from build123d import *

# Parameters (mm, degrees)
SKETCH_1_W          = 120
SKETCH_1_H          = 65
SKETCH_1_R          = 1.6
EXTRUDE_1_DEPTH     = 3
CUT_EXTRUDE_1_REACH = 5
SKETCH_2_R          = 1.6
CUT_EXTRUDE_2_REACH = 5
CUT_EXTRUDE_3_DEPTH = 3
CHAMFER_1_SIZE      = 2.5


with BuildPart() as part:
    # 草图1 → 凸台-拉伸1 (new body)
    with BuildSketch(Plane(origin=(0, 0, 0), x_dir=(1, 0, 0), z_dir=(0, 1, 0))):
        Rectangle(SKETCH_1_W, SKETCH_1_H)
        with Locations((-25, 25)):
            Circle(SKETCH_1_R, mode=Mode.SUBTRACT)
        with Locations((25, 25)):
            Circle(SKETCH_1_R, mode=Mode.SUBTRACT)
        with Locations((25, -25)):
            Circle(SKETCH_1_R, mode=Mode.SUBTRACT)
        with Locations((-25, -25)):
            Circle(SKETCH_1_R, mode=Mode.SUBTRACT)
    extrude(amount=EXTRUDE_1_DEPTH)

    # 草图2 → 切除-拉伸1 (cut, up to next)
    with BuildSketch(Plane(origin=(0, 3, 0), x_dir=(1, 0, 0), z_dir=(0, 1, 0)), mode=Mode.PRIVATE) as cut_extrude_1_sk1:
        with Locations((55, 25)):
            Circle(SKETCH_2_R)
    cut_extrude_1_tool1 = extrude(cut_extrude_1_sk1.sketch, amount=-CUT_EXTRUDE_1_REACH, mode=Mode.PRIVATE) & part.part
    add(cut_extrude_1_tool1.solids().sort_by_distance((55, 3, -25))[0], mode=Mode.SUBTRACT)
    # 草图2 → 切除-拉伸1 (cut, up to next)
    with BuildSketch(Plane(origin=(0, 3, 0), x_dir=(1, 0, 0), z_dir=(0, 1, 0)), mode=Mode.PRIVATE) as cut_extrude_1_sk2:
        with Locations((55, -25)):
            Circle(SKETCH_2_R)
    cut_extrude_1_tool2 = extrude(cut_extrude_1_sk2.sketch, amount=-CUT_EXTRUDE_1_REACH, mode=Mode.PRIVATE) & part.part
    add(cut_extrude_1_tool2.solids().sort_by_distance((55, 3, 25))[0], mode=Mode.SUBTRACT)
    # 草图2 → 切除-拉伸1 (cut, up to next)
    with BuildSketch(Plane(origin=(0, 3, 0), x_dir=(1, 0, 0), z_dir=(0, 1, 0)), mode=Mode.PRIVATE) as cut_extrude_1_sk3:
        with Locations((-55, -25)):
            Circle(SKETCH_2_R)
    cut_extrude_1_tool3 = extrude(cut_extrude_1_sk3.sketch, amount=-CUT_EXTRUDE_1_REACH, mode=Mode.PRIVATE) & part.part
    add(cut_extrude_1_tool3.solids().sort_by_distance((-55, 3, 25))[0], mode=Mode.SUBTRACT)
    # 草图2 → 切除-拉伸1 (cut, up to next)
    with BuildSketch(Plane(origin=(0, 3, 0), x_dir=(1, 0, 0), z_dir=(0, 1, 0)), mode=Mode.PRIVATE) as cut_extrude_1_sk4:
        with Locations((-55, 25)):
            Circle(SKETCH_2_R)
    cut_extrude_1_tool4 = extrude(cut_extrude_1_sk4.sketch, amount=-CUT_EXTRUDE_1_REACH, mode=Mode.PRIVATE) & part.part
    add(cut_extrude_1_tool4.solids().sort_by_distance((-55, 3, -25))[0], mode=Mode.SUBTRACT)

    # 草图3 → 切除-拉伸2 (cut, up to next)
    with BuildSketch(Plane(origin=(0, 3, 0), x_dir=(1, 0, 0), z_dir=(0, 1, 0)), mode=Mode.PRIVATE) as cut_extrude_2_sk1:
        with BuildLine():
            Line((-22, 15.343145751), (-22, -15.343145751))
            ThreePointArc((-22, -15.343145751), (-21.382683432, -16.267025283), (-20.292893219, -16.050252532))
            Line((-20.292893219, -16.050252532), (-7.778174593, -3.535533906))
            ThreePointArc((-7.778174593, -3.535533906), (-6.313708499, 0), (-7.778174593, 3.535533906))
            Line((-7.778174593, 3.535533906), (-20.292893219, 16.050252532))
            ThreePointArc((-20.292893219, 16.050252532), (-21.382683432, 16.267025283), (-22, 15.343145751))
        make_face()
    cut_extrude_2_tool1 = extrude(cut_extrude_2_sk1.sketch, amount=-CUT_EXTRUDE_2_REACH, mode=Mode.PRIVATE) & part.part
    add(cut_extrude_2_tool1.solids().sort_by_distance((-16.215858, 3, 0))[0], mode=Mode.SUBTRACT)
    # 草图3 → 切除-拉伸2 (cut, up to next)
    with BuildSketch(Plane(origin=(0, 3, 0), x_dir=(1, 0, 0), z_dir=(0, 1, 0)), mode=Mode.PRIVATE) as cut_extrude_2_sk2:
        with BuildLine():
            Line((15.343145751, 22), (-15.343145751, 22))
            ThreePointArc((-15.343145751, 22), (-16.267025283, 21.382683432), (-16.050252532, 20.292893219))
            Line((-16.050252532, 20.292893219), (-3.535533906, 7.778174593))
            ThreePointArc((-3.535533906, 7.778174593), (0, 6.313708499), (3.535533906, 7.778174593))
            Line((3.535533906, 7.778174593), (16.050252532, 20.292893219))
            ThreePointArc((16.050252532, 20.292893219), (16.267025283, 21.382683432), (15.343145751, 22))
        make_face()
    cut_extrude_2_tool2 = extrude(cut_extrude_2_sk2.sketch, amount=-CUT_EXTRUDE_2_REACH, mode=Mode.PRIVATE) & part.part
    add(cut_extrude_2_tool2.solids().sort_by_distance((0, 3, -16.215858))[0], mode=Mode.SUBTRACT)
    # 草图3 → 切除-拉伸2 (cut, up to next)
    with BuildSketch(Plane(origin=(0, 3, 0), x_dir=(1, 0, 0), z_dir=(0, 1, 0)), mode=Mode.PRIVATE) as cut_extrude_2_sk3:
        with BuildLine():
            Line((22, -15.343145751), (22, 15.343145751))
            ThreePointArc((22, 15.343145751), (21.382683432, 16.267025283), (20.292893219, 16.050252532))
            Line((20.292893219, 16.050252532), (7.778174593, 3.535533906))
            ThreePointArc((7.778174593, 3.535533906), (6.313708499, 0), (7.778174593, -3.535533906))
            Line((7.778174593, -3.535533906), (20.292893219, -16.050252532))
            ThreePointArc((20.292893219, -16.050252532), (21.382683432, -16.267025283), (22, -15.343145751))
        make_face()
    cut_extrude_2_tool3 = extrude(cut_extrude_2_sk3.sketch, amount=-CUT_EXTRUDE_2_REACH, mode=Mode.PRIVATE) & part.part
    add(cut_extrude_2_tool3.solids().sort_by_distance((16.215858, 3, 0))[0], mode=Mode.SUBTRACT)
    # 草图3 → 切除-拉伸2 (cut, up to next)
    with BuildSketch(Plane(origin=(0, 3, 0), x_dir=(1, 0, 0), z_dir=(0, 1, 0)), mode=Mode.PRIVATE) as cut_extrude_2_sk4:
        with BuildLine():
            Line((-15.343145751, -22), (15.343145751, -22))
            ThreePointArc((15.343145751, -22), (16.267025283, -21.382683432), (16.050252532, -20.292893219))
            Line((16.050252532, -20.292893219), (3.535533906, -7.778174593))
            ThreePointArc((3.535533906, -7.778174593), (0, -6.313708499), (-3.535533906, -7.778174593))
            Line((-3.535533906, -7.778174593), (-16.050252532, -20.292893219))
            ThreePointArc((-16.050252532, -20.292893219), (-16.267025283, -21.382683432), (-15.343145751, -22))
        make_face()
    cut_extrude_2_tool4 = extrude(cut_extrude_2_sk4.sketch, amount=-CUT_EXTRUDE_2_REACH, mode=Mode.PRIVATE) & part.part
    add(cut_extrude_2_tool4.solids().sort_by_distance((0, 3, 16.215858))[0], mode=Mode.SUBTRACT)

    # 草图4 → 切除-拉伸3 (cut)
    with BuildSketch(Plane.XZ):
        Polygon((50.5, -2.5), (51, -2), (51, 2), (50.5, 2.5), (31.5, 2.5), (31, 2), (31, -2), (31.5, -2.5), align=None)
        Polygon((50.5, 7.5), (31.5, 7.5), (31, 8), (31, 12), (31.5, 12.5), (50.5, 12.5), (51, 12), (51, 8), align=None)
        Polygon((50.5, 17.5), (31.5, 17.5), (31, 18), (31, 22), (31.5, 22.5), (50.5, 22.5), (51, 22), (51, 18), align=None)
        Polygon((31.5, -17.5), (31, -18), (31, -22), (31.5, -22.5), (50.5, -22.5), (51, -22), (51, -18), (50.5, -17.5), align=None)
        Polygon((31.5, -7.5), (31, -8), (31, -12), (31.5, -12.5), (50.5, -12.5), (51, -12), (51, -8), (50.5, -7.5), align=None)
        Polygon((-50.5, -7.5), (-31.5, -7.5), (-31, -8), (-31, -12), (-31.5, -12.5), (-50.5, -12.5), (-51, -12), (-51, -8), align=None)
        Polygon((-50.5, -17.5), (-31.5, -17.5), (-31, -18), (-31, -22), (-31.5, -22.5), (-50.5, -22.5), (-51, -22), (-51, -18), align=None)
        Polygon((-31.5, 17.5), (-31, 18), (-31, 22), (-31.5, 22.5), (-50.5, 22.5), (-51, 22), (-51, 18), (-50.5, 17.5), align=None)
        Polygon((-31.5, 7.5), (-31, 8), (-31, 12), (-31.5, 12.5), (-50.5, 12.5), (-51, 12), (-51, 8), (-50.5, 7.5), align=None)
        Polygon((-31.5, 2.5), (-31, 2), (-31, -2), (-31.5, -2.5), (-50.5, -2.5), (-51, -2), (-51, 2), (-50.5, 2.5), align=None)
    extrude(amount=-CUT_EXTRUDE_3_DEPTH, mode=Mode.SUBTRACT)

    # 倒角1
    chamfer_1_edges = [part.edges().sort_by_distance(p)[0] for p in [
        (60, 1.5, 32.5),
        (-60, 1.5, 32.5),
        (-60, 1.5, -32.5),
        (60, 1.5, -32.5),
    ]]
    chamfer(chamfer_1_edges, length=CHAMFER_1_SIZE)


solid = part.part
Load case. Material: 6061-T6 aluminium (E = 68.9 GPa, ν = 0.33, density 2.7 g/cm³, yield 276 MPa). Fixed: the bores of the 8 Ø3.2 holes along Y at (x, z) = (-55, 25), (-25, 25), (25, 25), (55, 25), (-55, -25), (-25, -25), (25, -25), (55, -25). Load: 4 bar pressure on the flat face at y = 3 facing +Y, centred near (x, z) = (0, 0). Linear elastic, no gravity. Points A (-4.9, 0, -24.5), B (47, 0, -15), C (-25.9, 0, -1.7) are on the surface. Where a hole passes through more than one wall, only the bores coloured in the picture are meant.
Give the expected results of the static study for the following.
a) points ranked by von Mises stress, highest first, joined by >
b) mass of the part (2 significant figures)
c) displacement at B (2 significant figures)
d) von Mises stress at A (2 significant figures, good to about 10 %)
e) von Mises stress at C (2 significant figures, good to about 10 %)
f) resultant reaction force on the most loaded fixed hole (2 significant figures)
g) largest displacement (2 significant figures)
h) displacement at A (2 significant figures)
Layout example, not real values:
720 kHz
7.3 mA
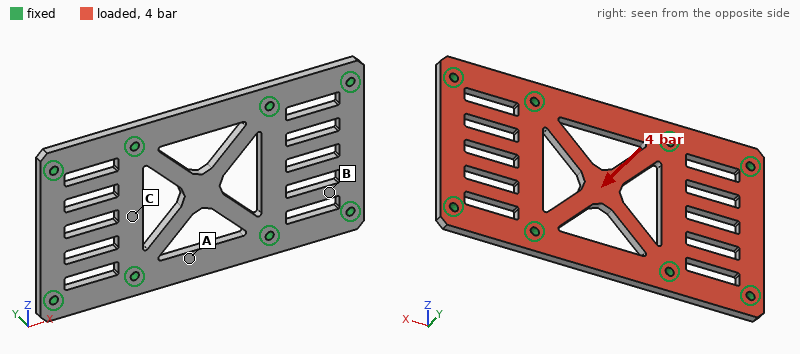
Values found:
C > A > B
45 g
0.027 mm
21 MPa
36 MPa
360 N
0.10 mm
0.036 mm
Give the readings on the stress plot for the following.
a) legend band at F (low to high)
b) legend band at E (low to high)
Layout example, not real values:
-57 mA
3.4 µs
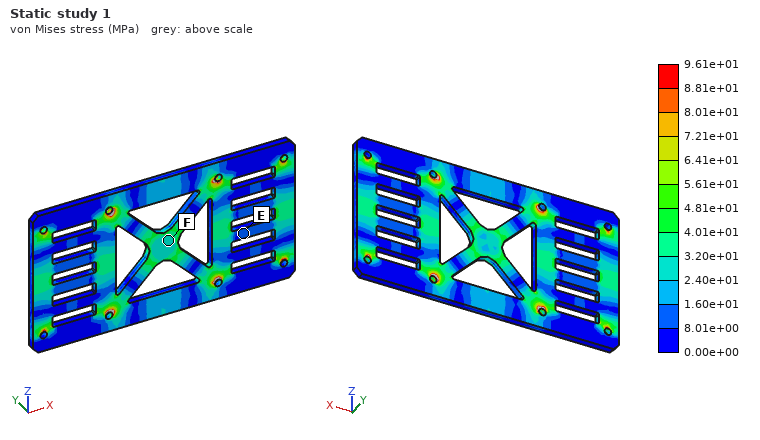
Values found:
2.40e+01 to 3.20e+01 MPa
8.01e+00 to 1.60e+01 MPa
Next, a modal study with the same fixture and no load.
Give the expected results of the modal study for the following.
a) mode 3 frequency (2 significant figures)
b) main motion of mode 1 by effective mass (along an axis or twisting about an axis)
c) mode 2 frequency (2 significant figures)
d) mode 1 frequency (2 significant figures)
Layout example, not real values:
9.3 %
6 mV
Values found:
5300 Hz
along Y
5300 Hz
4200 Hz
